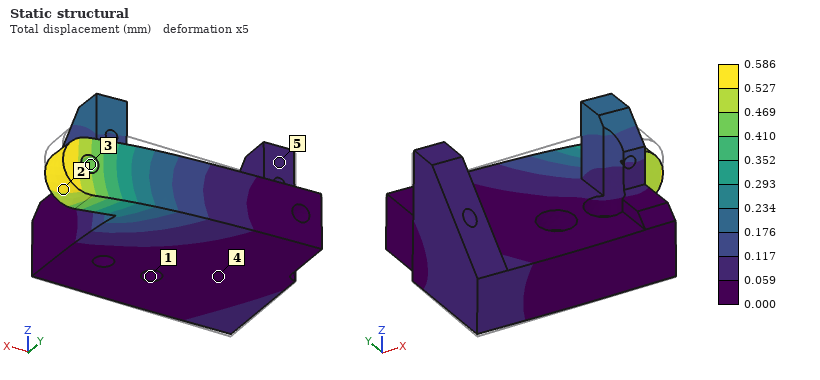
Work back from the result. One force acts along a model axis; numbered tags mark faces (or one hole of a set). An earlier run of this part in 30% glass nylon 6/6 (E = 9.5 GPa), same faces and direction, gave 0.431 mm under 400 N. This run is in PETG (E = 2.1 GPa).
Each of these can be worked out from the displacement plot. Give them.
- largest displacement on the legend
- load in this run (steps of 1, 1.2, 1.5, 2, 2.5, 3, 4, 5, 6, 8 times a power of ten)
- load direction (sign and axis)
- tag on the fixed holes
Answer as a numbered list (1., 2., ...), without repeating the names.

1. 0.586 mm
2. 120 N
3. -Z
4. 1
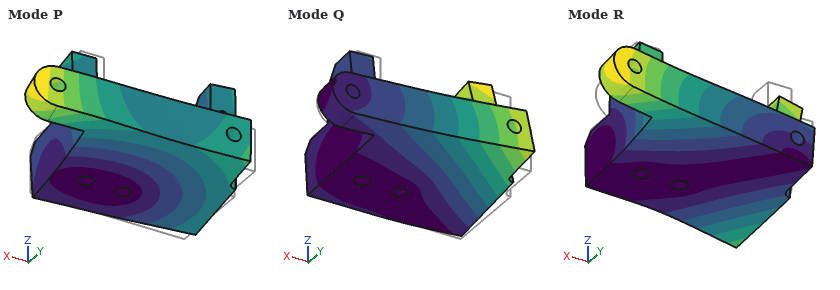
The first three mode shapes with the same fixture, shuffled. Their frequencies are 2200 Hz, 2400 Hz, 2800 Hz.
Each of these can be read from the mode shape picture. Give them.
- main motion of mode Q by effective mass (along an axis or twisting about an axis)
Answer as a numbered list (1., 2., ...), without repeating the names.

1. along Z
